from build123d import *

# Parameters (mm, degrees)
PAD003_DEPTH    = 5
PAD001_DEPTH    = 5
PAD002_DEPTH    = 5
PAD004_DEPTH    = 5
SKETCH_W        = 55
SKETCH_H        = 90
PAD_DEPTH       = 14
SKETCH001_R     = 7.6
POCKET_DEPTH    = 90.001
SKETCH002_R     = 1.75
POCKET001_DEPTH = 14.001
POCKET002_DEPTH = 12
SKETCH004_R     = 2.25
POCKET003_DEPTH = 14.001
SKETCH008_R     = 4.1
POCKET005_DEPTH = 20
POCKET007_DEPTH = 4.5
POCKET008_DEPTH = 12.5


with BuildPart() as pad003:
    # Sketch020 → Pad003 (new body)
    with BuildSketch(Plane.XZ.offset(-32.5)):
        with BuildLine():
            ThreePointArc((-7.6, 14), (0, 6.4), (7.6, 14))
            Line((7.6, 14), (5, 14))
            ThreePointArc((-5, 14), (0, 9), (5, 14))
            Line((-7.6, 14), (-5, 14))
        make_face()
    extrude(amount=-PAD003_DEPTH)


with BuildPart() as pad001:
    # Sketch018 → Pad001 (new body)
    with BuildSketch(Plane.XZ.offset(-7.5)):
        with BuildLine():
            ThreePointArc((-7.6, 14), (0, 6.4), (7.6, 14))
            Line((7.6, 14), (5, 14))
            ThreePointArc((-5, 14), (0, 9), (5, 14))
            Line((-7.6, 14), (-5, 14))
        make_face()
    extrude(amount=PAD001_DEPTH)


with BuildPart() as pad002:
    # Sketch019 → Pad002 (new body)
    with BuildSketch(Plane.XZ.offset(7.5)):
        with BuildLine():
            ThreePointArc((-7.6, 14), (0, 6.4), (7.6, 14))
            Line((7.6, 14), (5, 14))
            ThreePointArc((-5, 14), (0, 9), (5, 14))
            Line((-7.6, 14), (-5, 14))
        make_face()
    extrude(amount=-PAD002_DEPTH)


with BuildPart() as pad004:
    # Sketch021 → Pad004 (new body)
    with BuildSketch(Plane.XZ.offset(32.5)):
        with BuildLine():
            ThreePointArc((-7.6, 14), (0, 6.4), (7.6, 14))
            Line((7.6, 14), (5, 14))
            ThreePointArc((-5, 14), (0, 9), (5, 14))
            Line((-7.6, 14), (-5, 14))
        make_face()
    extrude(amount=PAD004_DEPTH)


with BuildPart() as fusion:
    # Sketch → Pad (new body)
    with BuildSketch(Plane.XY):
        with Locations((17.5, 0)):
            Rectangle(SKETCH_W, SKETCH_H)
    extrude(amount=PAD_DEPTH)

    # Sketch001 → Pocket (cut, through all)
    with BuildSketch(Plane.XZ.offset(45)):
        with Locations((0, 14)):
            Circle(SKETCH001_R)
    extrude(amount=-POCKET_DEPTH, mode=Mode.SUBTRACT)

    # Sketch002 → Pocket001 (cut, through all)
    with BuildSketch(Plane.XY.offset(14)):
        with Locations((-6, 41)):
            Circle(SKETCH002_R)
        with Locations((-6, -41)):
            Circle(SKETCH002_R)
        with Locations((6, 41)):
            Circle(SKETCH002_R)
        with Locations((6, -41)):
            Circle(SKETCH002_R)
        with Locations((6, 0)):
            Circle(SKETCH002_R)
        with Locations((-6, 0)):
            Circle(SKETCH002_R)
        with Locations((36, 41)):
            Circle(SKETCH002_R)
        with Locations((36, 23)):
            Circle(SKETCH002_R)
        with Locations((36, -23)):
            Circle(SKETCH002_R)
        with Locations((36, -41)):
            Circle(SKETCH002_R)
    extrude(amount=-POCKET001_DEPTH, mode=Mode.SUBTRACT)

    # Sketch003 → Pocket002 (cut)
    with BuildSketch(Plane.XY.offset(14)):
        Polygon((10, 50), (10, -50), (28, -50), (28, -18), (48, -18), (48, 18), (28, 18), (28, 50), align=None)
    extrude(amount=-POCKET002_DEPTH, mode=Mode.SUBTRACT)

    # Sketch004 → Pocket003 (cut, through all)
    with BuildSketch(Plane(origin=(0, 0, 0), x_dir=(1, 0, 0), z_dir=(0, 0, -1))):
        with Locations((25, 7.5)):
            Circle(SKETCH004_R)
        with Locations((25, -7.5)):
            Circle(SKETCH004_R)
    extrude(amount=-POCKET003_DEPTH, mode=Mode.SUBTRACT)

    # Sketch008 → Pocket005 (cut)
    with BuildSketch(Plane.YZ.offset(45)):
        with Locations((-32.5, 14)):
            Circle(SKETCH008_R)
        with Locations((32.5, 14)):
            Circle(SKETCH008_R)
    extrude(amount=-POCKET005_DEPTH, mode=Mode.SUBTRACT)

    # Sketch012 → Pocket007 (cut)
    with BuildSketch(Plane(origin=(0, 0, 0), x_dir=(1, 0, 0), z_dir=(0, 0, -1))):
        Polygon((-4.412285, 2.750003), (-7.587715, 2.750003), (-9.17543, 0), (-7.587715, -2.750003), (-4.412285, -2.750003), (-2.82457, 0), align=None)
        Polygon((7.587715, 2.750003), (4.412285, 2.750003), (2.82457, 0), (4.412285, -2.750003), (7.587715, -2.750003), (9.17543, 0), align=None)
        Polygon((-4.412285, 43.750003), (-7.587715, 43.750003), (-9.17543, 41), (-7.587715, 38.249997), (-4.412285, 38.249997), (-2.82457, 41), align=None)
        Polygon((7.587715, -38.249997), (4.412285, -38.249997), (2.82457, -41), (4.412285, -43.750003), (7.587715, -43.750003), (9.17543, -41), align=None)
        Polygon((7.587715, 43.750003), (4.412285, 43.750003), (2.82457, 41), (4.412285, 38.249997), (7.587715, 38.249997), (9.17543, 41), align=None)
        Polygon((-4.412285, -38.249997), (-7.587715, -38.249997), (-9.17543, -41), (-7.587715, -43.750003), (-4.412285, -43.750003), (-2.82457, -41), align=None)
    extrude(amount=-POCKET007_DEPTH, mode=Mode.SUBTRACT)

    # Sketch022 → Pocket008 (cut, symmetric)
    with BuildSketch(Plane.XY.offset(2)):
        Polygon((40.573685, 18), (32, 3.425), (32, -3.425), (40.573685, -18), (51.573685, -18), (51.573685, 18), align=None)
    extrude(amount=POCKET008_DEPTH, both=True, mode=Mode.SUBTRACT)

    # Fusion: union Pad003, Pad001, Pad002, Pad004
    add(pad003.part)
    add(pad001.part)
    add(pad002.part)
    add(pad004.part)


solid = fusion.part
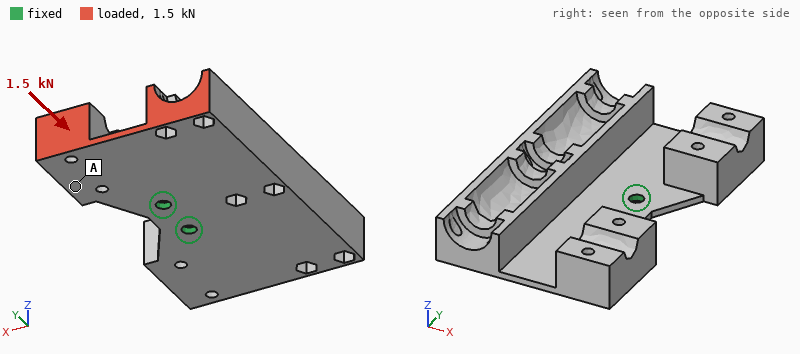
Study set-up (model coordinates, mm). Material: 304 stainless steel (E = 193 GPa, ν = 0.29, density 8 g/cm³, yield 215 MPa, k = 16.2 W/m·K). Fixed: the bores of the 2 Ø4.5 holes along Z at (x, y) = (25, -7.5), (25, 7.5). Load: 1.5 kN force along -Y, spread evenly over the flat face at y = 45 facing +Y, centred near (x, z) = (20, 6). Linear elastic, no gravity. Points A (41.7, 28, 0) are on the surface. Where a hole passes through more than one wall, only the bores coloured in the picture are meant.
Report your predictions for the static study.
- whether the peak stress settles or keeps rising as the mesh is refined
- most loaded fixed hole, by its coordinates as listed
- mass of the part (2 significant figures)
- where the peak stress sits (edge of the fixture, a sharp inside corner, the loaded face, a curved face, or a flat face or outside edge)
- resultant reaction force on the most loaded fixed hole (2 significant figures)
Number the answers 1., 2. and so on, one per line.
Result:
1. keeps rising
2. (25, 7.5)
3. 260 g
4. edge of the fixture
5. 1.2 kN
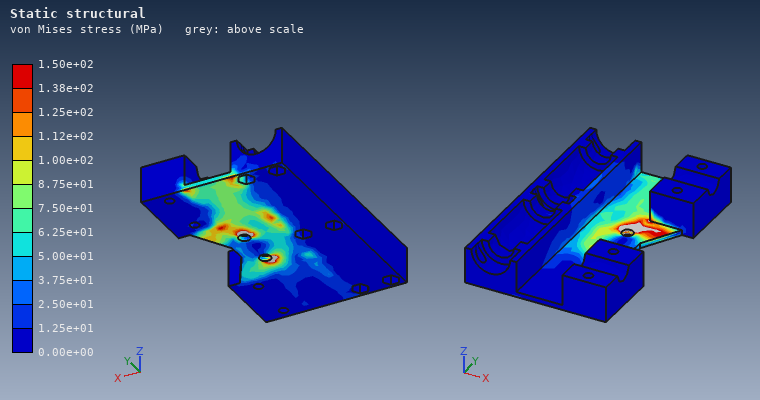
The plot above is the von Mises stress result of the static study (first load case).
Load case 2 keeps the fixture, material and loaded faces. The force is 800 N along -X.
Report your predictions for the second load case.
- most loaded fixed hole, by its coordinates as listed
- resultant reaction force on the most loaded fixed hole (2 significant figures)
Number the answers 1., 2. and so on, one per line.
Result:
1. (25, 7.5)
2. 2.2 kN
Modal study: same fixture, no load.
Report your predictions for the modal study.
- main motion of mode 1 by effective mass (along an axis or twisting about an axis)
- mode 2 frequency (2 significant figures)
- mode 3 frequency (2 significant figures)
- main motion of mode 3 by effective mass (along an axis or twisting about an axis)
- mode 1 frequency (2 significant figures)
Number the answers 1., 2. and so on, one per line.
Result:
1. along Z
2. 610 Hz
3. 880 Hz
4. along Z
5. 500 Hz
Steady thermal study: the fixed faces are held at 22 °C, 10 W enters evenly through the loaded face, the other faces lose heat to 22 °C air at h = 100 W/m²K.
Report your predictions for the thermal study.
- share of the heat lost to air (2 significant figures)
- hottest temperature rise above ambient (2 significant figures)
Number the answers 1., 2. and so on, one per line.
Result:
1. 96 %
2. 35 K
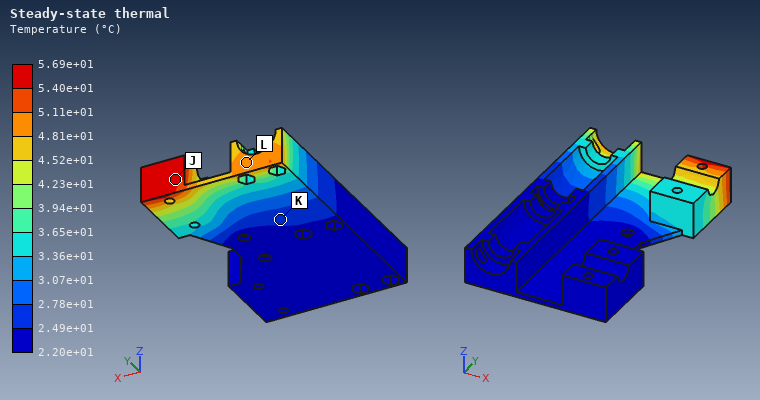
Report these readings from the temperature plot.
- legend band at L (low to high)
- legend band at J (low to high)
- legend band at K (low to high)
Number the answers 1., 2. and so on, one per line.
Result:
1. 4.81e+01 to 5.11e+01 °C
2. 5.40e+01 to 5.69e+01 °C
3. 2.49e+01 to 2.78e+01 °C
